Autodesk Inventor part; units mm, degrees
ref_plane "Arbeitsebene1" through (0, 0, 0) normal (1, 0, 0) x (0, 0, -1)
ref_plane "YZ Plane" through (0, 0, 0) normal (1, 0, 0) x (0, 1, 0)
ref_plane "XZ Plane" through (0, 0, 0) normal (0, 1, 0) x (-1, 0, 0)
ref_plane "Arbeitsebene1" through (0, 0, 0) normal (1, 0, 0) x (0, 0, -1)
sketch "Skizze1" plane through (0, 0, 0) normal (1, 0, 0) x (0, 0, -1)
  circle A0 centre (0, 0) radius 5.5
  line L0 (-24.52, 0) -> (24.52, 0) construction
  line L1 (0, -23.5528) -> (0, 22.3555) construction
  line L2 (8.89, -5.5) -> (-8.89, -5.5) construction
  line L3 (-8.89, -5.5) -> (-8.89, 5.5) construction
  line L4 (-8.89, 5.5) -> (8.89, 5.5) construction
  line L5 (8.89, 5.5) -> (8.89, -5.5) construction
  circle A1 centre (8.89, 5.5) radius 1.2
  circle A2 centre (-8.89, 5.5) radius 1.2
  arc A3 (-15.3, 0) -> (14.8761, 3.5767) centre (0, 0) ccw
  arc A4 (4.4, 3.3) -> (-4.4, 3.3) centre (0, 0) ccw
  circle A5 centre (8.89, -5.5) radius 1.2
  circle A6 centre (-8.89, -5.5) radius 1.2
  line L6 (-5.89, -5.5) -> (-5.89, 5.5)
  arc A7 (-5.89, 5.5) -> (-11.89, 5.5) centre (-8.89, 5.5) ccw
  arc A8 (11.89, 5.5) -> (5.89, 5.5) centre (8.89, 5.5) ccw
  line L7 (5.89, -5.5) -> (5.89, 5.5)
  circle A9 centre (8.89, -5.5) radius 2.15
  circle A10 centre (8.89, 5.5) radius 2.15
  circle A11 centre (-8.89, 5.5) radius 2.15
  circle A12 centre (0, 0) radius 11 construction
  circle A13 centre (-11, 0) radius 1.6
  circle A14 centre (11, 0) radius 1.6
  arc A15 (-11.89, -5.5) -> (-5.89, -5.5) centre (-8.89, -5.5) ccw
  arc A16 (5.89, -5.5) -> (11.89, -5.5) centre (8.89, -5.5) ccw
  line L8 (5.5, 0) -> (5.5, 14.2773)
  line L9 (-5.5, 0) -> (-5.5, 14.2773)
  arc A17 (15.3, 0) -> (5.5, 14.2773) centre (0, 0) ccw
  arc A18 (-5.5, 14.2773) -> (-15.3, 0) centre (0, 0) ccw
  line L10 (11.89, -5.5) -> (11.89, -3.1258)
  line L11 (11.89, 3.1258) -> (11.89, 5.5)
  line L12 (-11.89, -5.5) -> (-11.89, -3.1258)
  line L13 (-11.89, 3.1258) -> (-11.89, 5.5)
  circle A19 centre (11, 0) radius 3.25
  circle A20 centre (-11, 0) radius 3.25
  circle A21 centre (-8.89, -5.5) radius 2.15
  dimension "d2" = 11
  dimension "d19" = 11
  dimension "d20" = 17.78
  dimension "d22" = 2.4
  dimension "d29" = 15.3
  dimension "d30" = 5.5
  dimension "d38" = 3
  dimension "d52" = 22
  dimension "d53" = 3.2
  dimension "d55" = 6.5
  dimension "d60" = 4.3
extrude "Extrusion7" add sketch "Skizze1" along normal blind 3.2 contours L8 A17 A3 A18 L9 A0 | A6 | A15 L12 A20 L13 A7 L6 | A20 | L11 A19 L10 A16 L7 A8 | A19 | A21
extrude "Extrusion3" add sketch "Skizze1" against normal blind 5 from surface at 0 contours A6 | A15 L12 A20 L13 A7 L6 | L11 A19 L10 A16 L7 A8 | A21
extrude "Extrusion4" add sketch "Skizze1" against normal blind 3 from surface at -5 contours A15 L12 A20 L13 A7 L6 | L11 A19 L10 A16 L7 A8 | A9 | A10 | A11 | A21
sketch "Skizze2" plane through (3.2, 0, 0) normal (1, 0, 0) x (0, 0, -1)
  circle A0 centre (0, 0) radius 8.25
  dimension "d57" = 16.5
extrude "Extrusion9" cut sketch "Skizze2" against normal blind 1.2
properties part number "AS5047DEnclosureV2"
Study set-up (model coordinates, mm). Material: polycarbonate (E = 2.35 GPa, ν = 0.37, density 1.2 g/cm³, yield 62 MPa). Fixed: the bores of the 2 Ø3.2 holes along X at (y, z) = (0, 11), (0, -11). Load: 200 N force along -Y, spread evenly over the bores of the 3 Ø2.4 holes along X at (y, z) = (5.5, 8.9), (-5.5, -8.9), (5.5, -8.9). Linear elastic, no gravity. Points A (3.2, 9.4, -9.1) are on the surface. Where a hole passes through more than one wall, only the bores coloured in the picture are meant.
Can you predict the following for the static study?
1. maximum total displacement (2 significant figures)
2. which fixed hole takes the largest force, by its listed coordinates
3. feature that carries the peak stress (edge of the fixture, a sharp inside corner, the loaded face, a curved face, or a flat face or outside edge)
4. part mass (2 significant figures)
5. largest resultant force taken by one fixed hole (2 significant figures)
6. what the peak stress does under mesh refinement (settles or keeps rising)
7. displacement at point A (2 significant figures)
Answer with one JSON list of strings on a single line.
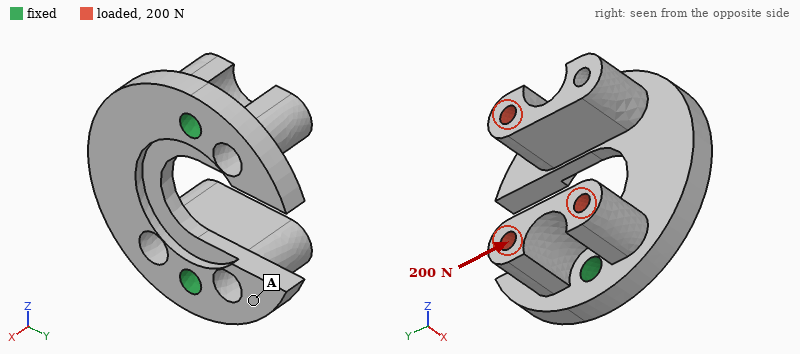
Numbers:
["0.45 mm", "(0, -11)", "edge of the fixture", "2.7 g", "130 N", "keeps rising", "0.25 mm"]
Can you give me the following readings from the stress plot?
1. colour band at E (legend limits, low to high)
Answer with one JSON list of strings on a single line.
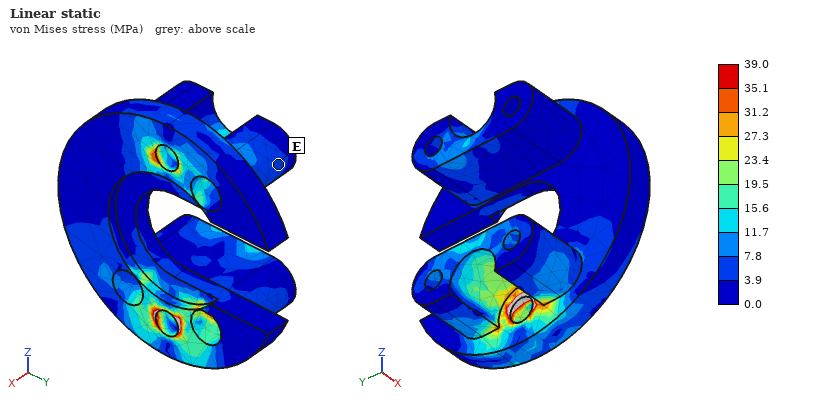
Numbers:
["3.9 to 7.8 MPa"]
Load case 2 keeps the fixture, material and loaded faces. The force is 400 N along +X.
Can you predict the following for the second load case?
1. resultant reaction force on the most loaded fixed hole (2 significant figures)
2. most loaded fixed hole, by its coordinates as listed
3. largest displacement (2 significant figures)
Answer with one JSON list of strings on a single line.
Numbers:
["260 N", "(0, -11)", "0.30 mm"]
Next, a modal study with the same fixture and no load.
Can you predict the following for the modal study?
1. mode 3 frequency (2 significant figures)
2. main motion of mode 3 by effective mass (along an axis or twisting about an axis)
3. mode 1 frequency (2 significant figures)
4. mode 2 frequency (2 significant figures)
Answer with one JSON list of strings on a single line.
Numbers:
["5000 Hz", "along X", "3100 Hz", "4400 Hz"]
